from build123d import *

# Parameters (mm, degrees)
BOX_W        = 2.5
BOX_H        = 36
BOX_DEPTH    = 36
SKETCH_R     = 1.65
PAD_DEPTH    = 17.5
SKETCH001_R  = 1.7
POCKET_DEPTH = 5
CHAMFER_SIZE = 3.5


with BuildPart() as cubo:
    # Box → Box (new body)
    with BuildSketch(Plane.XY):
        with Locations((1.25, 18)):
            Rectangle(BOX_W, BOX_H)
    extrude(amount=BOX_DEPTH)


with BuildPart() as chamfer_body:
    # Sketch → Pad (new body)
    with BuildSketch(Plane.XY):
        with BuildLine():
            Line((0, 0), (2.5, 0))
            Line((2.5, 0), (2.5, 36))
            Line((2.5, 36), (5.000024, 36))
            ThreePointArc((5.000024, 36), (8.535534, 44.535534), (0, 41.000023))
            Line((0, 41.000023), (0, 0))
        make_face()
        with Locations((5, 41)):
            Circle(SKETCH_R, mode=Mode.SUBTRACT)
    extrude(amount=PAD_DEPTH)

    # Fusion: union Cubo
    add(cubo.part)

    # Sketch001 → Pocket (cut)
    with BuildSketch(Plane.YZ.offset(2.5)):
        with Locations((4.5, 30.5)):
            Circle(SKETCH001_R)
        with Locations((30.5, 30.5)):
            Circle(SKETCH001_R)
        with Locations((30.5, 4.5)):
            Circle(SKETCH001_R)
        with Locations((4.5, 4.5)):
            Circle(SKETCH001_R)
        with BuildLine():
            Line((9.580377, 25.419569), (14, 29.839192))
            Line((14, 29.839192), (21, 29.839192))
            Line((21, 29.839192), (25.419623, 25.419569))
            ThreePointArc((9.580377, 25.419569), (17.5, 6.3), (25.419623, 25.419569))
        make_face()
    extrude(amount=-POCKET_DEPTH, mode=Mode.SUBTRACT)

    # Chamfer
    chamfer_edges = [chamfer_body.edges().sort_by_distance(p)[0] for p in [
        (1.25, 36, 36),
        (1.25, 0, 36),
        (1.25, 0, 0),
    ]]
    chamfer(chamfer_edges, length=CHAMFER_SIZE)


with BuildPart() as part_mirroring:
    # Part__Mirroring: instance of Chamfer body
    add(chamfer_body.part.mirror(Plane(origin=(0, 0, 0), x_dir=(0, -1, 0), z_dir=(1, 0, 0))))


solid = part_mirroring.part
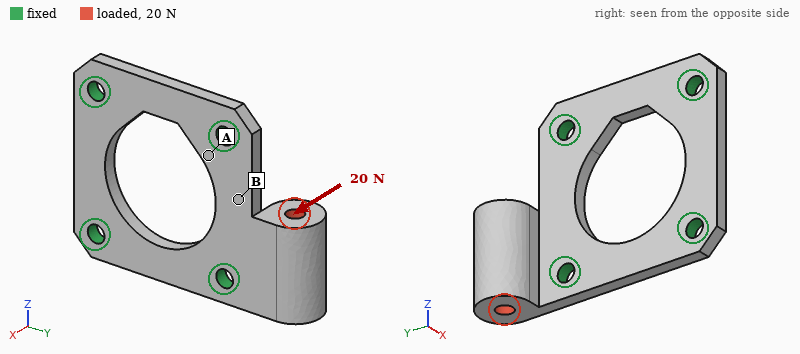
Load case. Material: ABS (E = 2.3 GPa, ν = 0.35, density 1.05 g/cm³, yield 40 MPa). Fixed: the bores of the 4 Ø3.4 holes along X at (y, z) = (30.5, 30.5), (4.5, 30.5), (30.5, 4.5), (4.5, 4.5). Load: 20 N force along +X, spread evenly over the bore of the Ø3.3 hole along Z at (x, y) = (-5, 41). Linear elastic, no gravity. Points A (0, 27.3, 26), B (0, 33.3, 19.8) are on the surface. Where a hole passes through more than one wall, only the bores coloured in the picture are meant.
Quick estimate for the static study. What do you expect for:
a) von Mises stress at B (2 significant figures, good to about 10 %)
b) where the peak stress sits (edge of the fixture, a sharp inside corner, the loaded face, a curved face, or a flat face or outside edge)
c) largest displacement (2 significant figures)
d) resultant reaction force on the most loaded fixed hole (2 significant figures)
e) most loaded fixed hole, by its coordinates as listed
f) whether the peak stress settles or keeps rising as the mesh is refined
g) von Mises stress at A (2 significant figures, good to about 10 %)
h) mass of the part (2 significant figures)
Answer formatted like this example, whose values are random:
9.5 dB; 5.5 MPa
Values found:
4.1 MPa; edge of the fixture; 0.27 mm; 18 N; (30.5, 4.5); keeps rising; 1.7 MPa; 3.6 g
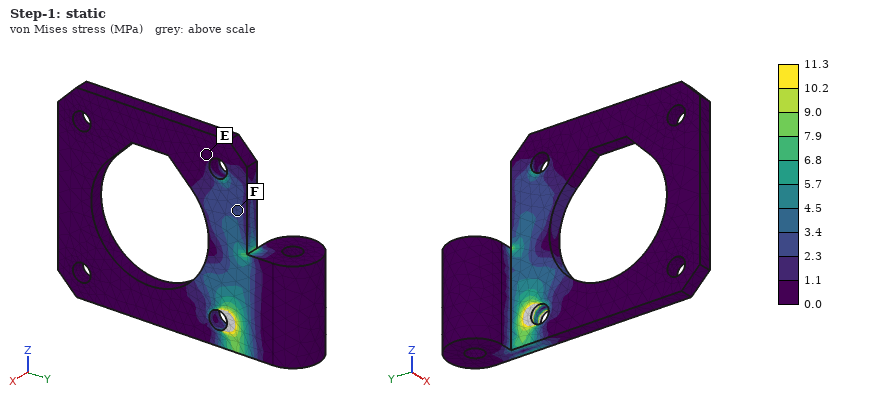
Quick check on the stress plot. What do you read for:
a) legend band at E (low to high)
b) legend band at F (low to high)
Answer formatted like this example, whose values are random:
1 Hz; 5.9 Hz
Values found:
0.0 to 1.1 MPa; 2.3 to 3.4 MPa
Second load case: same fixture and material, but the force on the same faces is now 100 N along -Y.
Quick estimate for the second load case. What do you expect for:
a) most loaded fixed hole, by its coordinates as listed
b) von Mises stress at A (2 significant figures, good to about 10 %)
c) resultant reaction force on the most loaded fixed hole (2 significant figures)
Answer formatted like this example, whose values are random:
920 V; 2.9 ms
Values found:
(30.5, 4.5); 3.0 MPa; 84 N
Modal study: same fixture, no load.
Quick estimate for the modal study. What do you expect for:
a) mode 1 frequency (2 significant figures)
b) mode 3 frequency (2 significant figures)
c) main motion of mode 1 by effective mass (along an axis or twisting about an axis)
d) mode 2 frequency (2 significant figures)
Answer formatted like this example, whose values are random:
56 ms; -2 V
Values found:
1400 Hz; 5600 Hz; along X; 3200 Hz
